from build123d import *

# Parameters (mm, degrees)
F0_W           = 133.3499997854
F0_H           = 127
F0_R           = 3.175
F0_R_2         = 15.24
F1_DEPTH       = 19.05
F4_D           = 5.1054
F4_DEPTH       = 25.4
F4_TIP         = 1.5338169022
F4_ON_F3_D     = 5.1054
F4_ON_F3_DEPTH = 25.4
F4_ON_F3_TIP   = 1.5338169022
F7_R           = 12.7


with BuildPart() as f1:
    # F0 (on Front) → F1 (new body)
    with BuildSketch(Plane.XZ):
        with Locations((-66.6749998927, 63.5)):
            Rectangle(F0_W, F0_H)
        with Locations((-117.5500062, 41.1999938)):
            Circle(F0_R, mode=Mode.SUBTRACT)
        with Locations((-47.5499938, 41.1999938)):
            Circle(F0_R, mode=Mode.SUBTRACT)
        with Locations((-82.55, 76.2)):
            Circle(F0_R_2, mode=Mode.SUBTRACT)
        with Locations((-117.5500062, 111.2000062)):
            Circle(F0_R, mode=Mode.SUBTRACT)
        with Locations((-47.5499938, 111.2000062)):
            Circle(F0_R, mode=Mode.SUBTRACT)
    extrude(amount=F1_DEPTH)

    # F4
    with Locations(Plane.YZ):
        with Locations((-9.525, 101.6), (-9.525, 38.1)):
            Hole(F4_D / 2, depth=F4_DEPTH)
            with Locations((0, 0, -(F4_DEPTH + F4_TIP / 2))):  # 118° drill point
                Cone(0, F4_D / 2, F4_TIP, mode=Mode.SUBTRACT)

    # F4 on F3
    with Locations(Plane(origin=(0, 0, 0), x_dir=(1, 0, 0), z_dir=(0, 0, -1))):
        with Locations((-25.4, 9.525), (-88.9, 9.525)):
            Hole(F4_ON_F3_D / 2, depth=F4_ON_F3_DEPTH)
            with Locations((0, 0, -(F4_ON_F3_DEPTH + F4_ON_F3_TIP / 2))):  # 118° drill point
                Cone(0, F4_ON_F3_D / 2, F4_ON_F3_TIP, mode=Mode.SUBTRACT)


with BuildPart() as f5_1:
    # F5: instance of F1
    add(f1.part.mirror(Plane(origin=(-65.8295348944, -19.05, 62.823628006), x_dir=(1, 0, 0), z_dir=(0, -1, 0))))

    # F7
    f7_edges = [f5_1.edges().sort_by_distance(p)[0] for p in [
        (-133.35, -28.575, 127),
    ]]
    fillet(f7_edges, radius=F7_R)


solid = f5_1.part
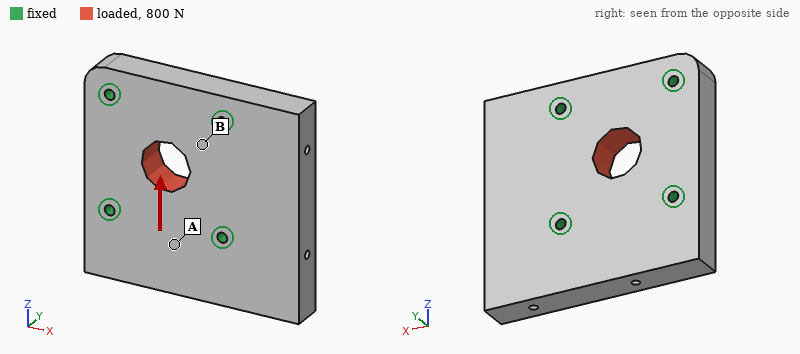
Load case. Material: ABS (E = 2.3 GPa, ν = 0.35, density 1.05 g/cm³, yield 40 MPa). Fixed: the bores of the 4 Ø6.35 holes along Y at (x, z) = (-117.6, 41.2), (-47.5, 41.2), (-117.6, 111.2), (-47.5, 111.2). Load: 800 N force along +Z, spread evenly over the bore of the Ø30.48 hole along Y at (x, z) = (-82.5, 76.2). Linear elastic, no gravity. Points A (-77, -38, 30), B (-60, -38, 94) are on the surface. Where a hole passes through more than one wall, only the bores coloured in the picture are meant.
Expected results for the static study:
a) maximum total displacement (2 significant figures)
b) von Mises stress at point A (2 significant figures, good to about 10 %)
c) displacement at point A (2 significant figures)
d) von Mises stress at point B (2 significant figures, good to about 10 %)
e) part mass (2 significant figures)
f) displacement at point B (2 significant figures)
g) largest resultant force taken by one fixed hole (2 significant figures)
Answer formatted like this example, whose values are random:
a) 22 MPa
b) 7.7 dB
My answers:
a) 11 µm
b) 0.16 MPa
c) 4.9 µm
d) 0.41 MPa
e) 320 g
f) 4.7 µm
g) 220 N
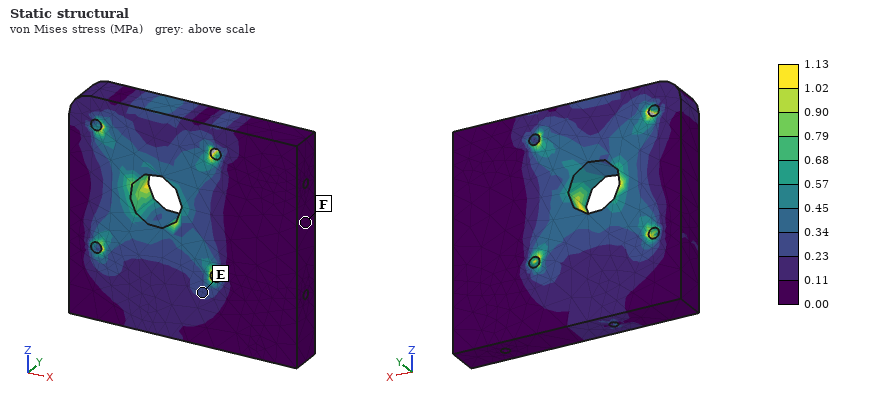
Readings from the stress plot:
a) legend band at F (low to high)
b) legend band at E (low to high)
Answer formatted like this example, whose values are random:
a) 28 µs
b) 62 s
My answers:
a) 0.00 to 0.11 MPa
b) 0.23 to 0.34 MPa
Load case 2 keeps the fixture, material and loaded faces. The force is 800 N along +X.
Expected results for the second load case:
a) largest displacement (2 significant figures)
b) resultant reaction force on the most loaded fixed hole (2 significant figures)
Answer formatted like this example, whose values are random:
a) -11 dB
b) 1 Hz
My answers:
a) 11 µm
b) 220 N
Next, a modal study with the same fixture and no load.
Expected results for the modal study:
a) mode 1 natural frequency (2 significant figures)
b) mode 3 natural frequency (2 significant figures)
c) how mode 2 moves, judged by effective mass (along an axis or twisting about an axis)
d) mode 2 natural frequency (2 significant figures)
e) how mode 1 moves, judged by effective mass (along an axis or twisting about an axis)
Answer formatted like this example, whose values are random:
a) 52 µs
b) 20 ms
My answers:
a) 1400 Hz
b) 2000 Hz
c) twisting about X
d) 1600 Hz
e) along Y
